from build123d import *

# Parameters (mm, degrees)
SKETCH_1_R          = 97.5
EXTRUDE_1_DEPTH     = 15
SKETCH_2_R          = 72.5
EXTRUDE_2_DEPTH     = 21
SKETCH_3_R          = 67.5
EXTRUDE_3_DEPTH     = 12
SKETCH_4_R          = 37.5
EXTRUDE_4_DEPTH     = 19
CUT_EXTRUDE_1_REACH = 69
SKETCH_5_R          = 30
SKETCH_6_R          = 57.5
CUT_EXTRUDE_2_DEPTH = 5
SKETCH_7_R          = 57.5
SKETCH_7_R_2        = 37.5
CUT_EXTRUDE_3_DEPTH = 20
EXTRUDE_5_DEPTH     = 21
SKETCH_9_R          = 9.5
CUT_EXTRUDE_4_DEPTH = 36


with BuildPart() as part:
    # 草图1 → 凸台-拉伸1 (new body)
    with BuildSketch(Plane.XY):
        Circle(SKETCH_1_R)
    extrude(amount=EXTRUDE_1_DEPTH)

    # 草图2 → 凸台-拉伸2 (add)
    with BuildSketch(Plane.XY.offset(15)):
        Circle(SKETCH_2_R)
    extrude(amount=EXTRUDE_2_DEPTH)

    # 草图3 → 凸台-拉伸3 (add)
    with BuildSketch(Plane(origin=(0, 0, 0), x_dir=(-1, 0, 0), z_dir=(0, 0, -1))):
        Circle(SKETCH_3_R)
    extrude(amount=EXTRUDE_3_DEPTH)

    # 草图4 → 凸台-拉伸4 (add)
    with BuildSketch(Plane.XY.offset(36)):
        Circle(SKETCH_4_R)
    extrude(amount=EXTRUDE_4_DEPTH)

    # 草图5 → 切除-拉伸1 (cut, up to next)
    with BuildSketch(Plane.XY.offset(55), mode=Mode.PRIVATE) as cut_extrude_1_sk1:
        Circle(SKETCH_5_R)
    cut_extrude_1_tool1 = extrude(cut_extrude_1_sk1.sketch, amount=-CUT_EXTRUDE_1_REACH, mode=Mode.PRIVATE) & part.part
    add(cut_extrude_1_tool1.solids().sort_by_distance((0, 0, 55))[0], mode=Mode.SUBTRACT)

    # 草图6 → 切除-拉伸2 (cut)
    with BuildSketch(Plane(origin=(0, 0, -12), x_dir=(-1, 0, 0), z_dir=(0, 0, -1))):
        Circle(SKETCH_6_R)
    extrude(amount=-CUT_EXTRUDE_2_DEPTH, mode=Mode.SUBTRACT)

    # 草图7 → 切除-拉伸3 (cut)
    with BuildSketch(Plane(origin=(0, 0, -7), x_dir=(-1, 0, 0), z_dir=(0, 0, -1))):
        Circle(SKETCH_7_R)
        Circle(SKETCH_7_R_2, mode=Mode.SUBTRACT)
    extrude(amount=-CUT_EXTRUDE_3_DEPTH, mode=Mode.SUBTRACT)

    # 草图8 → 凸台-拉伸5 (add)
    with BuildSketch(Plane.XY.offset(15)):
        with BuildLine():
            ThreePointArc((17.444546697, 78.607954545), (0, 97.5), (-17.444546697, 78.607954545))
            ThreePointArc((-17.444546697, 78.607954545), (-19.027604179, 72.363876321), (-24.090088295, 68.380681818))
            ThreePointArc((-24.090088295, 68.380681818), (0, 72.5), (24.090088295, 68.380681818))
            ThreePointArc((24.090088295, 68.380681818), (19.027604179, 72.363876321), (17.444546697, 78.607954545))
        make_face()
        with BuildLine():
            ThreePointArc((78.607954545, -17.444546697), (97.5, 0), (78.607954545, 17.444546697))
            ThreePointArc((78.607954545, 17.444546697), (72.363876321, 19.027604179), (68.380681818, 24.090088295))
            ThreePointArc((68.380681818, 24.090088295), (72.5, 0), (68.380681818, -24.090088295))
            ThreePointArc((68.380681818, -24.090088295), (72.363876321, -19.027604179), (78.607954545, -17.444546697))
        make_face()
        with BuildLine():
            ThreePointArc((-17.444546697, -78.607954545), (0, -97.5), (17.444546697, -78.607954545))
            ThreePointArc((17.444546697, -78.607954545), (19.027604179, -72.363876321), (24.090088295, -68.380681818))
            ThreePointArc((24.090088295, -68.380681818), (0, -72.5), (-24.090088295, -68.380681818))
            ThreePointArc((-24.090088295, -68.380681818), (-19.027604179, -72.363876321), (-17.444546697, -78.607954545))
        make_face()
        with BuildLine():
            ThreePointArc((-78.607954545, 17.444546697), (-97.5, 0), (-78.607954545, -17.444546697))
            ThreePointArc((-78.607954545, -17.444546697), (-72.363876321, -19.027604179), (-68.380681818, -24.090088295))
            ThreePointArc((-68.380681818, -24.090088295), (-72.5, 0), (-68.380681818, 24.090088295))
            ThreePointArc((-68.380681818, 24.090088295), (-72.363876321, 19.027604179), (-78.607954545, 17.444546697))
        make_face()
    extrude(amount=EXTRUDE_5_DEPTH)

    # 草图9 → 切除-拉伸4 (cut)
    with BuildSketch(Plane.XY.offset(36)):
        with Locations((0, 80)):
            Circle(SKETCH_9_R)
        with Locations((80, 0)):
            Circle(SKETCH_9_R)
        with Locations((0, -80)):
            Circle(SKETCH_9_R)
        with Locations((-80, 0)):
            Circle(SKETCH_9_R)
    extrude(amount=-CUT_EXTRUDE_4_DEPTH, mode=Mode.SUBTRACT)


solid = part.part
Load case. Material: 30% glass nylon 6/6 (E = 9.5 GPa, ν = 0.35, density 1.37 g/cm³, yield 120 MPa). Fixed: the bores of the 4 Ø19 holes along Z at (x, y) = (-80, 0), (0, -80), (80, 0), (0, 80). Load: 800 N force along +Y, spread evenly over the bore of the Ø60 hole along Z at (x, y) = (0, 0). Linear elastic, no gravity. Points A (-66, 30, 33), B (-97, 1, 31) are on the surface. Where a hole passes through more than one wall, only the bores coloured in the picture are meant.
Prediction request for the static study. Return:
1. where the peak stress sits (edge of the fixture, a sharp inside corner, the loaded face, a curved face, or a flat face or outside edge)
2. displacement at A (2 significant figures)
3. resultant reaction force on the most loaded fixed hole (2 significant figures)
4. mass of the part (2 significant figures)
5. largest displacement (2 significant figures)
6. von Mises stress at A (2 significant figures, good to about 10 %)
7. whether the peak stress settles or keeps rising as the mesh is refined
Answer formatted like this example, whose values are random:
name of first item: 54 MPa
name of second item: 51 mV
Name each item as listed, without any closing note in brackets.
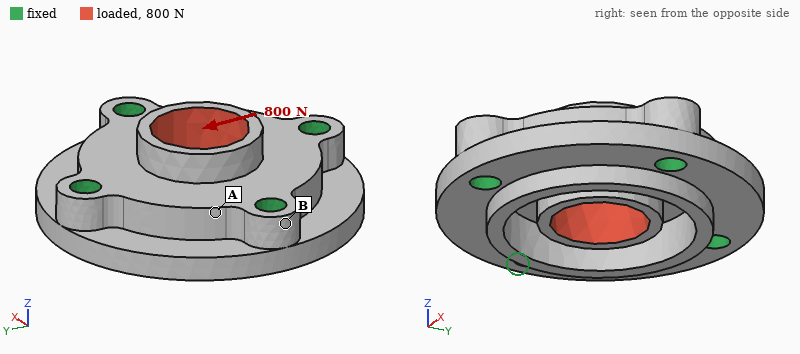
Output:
where the peak stress sits: edge of the fixture
displacement at A: 0.66 µm
resultant reaction force on the most loaded fixed hole: 260 N
mass of the part: 1000 g
largest displacement: 3.3 µm
von Mises stress at A: 0.11 MPa
whether the peak stress settles or keeps rising as the mesh is refined: keeps rising
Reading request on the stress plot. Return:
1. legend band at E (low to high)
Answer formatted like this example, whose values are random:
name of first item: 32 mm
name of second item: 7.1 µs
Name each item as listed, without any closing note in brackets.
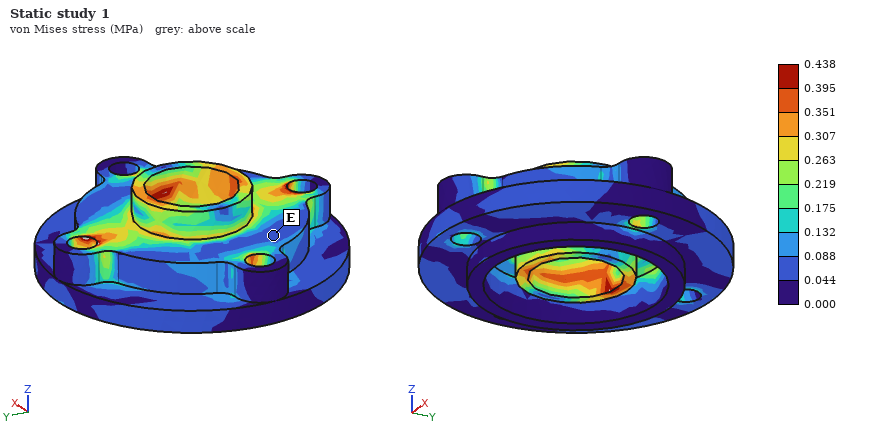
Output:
legend band at E: 0.044 to 0.088 MPa
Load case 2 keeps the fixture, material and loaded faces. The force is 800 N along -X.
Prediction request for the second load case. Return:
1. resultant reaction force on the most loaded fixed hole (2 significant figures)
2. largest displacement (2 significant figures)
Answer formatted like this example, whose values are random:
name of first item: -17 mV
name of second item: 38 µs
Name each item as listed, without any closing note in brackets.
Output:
resultant reaction force on the most loaded fixed hole: 260 N
largest displacement: 3.2 µm
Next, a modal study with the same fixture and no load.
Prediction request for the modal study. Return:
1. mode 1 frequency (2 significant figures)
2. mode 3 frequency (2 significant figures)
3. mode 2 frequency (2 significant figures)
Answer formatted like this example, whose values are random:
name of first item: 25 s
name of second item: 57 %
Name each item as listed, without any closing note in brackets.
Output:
mode 1 frequency: 3800 Hz
mode 3 frequency: 4100 Hz
mode 2 frequency: 4100 Hz
